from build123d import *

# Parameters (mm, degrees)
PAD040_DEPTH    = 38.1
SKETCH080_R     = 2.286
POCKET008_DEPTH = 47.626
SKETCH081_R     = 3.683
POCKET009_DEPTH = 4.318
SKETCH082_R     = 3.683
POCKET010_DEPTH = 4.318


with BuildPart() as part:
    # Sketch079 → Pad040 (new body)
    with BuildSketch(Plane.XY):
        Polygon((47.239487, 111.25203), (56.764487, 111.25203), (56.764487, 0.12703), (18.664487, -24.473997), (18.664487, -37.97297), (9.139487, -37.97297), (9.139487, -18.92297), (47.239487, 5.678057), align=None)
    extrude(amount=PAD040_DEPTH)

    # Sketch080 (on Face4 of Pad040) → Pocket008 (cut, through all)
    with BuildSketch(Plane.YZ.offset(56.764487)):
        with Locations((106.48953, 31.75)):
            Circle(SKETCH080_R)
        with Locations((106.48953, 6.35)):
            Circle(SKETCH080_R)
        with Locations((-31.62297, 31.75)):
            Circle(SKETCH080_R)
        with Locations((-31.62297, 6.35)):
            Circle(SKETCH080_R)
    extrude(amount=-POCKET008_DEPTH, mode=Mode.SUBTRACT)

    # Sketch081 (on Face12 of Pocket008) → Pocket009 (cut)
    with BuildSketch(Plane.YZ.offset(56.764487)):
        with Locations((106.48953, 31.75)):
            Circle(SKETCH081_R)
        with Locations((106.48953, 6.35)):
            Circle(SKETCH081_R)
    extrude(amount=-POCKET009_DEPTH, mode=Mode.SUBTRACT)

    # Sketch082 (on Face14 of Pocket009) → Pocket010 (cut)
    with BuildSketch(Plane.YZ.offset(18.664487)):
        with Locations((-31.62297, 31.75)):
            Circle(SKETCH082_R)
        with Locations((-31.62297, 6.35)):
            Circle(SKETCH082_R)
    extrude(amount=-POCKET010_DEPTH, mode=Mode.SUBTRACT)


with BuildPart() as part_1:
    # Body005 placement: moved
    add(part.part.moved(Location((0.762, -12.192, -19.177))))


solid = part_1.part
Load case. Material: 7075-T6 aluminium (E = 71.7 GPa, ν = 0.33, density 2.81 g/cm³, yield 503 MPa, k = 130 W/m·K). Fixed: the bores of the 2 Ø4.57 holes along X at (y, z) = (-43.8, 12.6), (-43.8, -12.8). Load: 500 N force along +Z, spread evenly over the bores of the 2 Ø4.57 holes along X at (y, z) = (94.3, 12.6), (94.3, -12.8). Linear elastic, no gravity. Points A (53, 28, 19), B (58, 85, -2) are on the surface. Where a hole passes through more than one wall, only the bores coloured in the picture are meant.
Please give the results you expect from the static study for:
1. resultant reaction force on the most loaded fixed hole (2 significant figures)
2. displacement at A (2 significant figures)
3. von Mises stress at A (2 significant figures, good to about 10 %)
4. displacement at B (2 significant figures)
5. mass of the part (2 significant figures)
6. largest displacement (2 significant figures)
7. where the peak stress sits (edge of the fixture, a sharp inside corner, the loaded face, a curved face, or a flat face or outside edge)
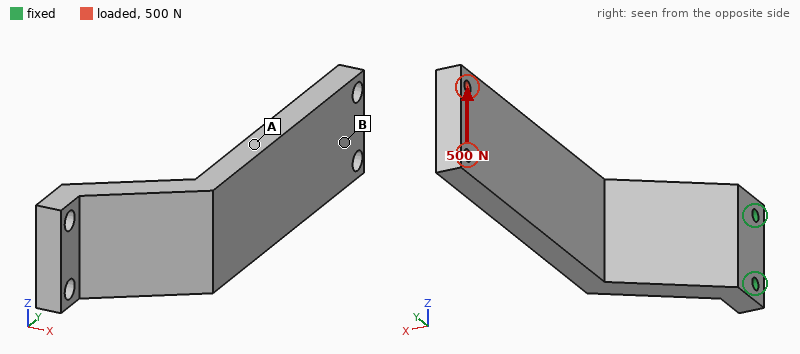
2.6 kN
0.27 mm
14 MPa
0.57 mm
170 g
0.71 mm
edge of the fixture
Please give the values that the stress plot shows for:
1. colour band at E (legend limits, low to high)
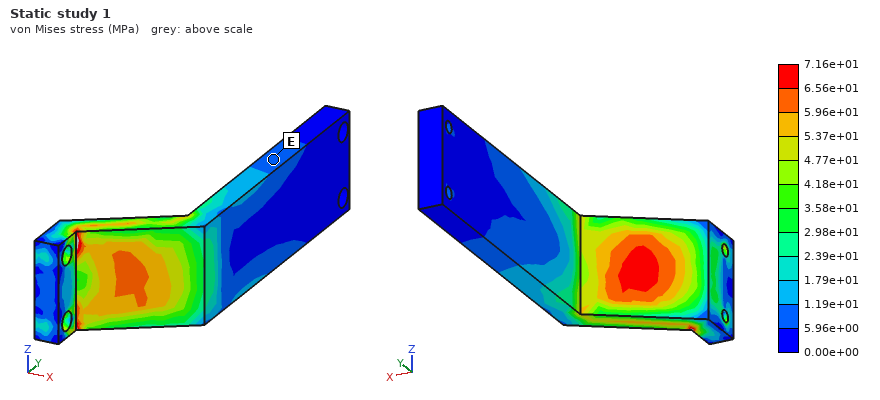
5.96e+00 to 1.19e+01 MPa
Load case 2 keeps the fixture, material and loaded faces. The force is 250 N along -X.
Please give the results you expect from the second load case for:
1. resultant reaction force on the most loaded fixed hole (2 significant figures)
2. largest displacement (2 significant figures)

190 N
1.8 mm
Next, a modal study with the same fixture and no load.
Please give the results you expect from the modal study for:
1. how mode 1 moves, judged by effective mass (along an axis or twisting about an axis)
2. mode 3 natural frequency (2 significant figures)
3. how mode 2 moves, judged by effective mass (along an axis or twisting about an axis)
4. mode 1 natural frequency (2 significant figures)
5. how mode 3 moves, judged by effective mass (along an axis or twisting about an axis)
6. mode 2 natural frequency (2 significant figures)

along X
1400 Hz
along Z
290 Hz
along Y
700 Hz
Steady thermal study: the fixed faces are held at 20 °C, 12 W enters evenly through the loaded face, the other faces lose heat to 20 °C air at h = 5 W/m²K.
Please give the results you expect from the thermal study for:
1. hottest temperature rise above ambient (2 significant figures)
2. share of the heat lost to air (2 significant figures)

39 K
13 %
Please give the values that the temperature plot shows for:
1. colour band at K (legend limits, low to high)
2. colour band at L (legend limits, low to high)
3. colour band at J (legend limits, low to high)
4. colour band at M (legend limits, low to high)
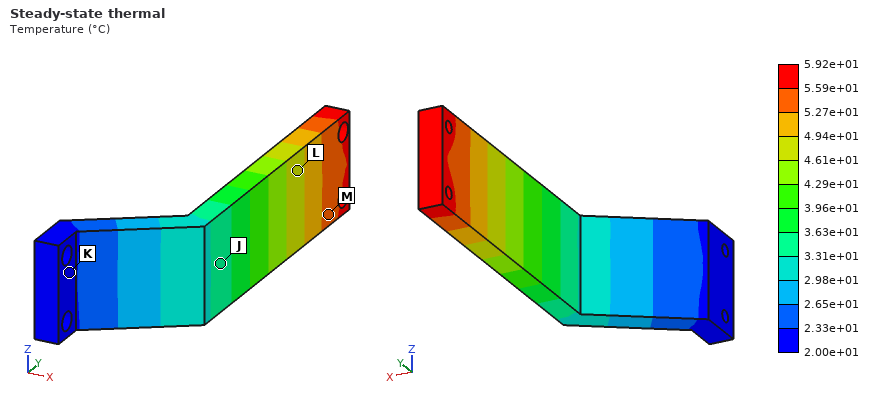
2.00e+01 to 2.33e+01 °C
4.61e+01 to 4.94e+01 °C
3.31e+01 to 3.63e+01 °C
5.27e+01 to 5.59e+01 °C
